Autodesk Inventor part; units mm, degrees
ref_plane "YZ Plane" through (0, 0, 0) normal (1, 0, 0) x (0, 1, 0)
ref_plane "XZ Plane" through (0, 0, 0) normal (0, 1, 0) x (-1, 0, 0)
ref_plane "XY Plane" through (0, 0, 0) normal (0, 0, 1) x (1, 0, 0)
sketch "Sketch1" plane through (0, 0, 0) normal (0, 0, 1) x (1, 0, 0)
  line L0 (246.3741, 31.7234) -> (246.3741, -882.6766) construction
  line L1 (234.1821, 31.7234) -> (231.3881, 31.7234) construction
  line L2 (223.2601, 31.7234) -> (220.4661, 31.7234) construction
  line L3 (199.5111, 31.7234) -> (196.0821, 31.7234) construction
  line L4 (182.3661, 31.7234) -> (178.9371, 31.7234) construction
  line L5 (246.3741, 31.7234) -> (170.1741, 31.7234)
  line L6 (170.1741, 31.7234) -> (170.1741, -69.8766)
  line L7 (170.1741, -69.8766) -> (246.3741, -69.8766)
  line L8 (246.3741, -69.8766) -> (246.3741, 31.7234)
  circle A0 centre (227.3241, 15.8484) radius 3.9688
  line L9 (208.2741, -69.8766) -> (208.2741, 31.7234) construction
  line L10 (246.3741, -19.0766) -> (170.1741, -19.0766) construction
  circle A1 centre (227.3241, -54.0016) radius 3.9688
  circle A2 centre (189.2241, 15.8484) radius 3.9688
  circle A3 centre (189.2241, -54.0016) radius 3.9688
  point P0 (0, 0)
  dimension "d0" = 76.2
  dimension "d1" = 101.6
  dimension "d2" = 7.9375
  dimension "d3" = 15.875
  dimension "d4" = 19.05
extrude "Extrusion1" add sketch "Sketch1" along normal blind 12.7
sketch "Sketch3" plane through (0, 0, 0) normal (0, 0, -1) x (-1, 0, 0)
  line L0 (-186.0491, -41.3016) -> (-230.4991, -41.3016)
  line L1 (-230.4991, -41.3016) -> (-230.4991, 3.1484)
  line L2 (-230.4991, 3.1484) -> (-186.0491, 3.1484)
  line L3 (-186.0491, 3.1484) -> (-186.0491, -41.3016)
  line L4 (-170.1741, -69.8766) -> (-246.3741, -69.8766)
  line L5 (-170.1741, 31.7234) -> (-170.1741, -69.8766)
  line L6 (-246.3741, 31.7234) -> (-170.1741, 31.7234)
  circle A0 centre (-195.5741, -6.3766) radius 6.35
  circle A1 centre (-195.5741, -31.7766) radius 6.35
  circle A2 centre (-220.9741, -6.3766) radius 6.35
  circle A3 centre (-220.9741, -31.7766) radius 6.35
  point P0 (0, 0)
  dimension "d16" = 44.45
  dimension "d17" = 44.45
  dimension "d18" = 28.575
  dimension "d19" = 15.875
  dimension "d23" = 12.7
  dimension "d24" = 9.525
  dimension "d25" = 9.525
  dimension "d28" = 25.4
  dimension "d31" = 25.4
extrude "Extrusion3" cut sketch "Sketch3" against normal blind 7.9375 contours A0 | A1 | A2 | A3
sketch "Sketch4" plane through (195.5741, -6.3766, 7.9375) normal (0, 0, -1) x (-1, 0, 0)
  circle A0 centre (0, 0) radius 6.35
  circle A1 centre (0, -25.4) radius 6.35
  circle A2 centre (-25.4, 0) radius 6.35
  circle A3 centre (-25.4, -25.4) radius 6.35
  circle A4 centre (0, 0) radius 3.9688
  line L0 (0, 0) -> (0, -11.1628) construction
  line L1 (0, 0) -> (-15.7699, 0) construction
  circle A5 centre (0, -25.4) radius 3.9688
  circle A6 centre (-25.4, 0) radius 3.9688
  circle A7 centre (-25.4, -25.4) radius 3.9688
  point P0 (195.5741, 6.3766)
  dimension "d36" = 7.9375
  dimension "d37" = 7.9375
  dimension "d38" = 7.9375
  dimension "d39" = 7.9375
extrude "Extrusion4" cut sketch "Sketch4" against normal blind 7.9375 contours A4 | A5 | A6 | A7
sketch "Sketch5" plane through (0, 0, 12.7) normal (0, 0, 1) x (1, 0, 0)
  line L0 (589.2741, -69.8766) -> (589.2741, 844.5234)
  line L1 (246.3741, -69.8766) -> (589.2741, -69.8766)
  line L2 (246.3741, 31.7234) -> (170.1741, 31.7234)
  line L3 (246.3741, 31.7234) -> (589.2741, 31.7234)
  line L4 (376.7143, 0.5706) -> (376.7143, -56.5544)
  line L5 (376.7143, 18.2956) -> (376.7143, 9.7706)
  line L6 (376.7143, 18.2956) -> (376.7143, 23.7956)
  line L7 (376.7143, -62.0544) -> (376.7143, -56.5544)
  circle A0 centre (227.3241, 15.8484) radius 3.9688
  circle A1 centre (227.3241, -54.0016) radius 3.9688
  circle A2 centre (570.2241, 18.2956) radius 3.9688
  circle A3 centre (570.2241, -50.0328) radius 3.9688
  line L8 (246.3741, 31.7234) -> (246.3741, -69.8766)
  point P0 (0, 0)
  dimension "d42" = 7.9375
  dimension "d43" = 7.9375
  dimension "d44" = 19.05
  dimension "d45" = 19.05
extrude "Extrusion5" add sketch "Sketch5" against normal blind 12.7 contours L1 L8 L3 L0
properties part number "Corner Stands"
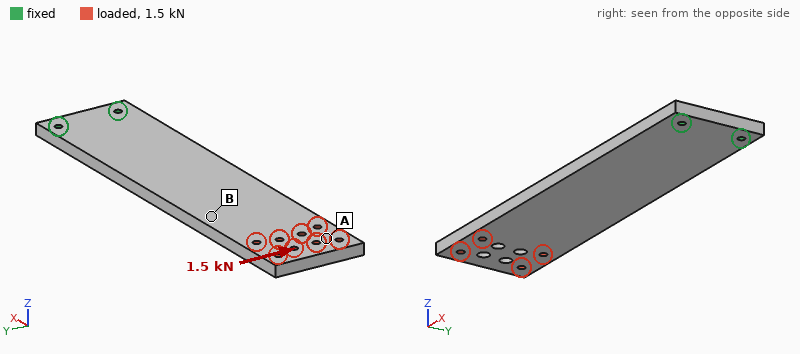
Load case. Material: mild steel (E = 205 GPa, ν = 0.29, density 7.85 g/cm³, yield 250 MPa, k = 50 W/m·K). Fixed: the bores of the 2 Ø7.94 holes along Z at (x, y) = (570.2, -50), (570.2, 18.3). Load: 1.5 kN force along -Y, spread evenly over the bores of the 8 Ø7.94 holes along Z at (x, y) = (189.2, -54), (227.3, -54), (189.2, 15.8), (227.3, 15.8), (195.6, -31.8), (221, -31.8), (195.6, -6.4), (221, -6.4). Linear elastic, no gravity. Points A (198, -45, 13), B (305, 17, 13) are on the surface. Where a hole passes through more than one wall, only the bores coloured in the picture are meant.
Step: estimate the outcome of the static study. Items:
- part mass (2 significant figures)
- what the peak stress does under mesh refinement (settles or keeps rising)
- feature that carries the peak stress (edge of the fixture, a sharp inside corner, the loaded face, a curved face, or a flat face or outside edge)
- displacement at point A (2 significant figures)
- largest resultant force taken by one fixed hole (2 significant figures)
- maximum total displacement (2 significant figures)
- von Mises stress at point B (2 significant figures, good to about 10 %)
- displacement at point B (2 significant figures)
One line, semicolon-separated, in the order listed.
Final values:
4.2 kg; keeps rising; edge of the fixture; 0.12 mm; 7.7 kN; 0.14 mm; 5.1 MPa; 0.075 mm
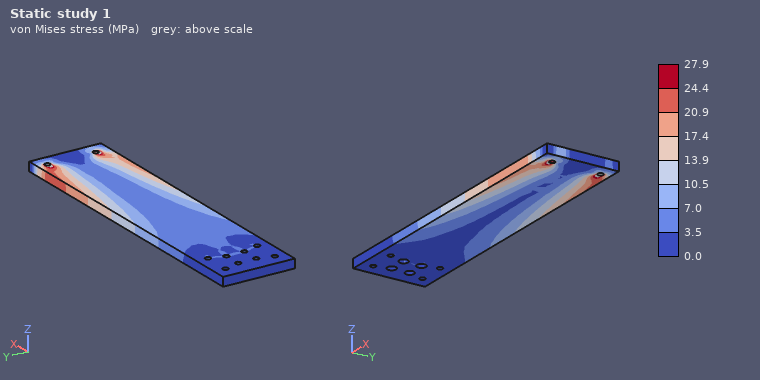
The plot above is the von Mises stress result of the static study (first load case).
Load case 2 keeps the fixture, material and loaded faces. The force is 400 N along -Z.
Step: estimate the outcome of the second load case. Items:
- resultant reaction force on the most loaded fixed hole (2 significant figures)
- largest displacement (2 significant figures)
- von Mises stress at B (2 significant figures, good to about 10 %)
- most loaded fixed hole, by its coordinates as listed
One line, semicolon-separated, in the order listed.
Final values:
250 N; 2.1 mm; 14 MPa; (570.2, -50)
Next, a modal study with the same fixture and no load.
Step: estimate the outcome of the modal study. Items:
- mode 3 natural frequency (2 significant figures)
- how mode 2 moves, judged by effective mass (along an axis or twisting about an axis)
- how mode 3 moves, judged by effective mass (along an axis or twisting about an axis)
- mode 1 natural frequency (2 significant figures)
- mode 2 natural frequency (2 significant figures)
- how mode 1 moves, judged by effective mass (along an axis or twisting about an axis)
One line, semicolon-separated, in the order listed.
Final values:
490 Hz; along Z; along Y; 66 Hz; 410 Hz; along Z
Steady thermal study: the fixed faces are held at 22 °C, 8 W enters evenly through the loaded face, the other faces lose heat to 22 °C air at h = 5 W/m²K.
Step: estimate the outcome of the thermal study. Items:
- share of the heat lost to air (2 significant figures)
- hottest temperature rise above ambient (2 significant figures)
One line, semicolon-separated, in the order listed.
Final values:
66 %; 24 K
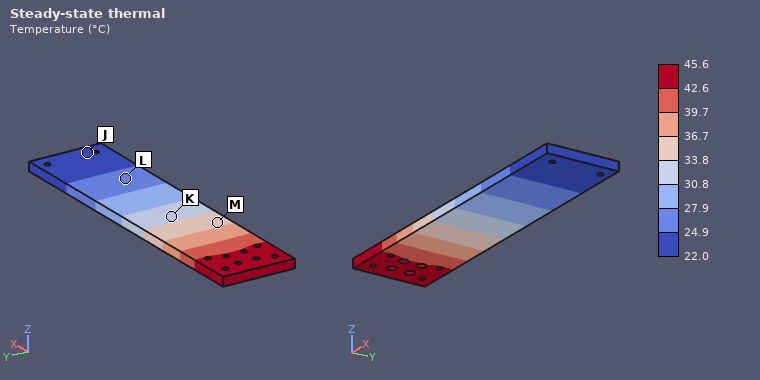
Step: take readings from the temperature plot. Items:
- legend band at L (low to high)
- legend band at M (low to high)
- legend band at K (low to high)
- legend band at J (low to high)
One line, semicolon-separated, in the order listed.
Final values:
24.9 to 27.9 °C; 33.8 to 36.7 °C; 30.8 to 33.8 °C; 22.0 to 24.9 °C
